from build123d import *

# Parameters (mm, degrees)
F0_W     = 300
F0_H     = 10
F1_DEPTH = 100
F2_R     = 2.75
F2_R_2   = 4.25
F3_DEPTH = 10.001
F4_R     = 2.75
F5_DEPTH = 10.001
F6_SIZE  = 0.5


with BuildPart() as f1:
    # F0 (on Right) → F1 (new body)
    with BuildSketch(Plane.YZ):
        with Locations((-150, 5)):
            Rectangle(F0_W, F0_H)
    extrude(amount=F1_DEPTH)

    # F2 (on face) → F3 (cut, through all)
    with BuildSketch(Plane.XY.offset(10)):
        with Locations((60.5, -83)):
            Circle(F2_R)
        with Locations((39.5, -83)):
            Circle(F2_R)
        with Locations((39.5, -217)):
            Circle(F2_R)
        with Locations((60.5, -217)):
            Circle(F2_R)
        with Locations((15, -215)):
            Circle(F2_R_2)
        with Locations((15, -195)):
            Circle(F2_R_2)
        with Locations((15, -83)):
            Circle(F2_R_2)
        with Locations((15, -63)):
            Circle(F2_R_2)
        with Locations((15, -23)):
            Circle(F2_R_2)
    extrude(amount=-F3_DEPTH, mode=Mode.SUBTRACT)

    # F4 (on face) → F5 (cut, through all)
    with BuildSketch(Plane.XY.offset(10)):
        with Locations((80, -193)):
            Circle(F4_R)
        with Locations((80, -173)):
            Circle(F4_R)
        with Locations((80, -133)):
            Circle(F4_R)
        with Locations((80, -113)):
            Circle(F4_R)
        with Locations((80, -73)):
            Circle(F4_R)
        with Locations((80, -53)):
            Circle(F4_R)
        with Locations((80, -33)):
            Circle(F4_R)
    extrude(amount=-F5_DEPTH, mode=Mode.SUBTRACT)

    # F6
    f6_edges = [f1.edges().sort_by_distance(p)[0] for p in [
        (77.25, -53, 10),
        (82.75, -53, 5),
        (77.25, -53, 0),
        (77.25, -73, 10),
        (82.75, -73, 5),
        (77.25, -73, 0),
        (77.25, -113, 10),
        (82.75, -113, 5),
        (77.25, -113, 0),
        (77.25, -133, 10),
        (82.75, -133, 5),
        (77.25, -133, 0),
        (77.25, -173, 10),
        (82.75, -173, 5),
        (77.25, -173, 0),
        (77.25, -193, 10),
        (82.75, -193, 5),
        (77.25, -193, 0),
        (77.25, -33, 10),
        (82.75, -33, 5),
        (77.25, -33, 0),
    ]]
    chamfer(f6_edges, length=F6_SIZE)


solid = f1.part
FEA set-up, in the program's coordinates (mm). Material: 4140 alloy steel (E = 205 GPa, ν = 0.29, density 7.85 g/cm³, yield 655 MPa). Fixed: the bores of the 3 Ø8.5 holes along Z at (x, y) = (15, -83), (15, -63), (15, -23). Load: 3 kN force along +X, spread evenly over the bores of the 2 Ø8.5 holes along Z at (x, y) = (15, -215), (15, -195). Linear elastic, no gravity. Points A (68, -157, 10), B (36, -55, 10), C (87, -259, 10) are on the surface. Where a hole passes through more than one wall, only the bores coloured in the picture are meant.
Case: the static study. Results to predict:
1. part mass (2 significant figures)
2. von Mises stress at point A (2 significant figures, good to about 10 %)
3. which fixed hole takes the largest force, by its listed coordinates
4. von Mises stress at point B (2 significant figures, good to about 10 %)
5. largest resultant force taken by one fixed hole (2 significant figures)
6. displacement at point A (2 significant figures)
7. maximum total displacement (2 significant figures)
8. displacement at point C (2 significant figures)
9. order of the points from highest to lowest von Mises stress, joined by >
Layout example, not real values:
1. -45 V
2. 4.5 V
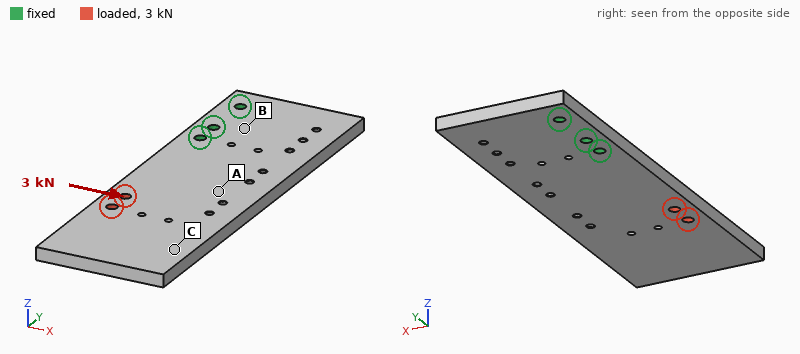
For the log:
1. 2.3 kg
2. 7.5 MPa
3. (15, -83)
4. 15 MPa
5. 8.4 kN
6. 26 µm
7. 72 µm
8. 59 µm
9. B > A > C
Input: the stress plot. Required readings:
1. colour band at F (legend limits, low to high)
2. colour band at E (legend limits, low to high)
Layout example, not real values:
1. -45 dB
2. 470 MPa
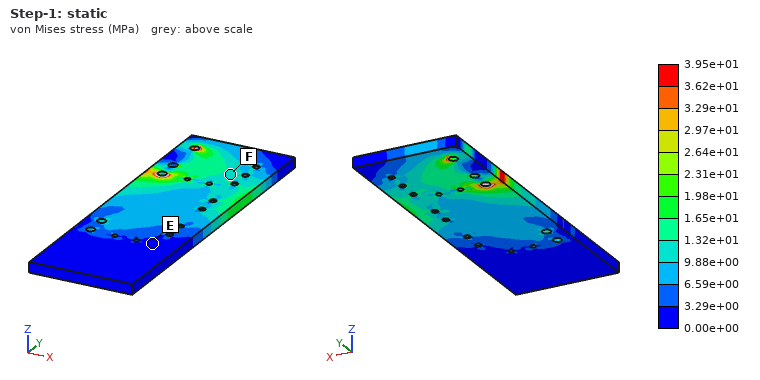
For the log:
1. 9.88e+00 to 1.32e+01 MPa
2. 0.00e+00 to 3.29e+00 MPa
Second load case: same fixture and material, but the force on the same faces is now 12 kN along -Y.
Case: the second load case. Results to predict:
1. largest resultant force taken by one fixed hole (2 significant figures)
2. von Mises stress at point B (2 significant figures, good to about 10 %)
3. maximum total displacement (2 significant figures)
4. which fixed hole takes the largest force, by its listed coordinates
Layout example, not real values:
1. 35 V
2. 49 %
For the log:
1. 9.1 kN
2. 5.7 MPa
3. 53 µm
4. (15, -83)
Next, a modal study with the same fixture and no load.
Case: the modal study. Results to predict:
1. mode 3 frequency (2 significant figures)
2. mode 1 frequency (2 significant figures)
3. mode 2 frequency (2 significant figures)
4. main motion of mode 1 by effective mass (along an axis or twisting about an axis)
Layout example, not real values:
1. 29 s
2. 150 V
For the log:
1. 970 Hz
2. 160 Hz
3. 600 Hz
4. along Z
